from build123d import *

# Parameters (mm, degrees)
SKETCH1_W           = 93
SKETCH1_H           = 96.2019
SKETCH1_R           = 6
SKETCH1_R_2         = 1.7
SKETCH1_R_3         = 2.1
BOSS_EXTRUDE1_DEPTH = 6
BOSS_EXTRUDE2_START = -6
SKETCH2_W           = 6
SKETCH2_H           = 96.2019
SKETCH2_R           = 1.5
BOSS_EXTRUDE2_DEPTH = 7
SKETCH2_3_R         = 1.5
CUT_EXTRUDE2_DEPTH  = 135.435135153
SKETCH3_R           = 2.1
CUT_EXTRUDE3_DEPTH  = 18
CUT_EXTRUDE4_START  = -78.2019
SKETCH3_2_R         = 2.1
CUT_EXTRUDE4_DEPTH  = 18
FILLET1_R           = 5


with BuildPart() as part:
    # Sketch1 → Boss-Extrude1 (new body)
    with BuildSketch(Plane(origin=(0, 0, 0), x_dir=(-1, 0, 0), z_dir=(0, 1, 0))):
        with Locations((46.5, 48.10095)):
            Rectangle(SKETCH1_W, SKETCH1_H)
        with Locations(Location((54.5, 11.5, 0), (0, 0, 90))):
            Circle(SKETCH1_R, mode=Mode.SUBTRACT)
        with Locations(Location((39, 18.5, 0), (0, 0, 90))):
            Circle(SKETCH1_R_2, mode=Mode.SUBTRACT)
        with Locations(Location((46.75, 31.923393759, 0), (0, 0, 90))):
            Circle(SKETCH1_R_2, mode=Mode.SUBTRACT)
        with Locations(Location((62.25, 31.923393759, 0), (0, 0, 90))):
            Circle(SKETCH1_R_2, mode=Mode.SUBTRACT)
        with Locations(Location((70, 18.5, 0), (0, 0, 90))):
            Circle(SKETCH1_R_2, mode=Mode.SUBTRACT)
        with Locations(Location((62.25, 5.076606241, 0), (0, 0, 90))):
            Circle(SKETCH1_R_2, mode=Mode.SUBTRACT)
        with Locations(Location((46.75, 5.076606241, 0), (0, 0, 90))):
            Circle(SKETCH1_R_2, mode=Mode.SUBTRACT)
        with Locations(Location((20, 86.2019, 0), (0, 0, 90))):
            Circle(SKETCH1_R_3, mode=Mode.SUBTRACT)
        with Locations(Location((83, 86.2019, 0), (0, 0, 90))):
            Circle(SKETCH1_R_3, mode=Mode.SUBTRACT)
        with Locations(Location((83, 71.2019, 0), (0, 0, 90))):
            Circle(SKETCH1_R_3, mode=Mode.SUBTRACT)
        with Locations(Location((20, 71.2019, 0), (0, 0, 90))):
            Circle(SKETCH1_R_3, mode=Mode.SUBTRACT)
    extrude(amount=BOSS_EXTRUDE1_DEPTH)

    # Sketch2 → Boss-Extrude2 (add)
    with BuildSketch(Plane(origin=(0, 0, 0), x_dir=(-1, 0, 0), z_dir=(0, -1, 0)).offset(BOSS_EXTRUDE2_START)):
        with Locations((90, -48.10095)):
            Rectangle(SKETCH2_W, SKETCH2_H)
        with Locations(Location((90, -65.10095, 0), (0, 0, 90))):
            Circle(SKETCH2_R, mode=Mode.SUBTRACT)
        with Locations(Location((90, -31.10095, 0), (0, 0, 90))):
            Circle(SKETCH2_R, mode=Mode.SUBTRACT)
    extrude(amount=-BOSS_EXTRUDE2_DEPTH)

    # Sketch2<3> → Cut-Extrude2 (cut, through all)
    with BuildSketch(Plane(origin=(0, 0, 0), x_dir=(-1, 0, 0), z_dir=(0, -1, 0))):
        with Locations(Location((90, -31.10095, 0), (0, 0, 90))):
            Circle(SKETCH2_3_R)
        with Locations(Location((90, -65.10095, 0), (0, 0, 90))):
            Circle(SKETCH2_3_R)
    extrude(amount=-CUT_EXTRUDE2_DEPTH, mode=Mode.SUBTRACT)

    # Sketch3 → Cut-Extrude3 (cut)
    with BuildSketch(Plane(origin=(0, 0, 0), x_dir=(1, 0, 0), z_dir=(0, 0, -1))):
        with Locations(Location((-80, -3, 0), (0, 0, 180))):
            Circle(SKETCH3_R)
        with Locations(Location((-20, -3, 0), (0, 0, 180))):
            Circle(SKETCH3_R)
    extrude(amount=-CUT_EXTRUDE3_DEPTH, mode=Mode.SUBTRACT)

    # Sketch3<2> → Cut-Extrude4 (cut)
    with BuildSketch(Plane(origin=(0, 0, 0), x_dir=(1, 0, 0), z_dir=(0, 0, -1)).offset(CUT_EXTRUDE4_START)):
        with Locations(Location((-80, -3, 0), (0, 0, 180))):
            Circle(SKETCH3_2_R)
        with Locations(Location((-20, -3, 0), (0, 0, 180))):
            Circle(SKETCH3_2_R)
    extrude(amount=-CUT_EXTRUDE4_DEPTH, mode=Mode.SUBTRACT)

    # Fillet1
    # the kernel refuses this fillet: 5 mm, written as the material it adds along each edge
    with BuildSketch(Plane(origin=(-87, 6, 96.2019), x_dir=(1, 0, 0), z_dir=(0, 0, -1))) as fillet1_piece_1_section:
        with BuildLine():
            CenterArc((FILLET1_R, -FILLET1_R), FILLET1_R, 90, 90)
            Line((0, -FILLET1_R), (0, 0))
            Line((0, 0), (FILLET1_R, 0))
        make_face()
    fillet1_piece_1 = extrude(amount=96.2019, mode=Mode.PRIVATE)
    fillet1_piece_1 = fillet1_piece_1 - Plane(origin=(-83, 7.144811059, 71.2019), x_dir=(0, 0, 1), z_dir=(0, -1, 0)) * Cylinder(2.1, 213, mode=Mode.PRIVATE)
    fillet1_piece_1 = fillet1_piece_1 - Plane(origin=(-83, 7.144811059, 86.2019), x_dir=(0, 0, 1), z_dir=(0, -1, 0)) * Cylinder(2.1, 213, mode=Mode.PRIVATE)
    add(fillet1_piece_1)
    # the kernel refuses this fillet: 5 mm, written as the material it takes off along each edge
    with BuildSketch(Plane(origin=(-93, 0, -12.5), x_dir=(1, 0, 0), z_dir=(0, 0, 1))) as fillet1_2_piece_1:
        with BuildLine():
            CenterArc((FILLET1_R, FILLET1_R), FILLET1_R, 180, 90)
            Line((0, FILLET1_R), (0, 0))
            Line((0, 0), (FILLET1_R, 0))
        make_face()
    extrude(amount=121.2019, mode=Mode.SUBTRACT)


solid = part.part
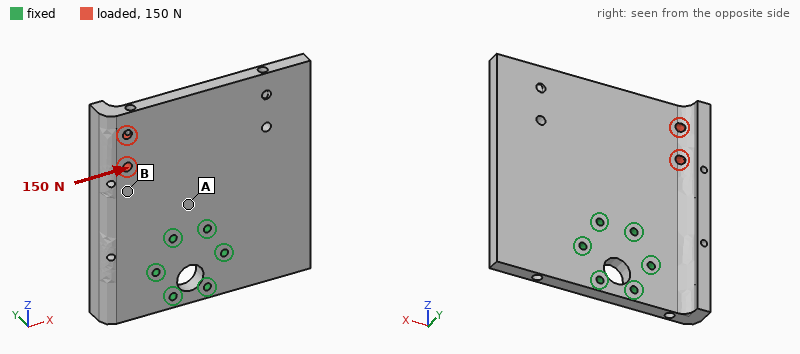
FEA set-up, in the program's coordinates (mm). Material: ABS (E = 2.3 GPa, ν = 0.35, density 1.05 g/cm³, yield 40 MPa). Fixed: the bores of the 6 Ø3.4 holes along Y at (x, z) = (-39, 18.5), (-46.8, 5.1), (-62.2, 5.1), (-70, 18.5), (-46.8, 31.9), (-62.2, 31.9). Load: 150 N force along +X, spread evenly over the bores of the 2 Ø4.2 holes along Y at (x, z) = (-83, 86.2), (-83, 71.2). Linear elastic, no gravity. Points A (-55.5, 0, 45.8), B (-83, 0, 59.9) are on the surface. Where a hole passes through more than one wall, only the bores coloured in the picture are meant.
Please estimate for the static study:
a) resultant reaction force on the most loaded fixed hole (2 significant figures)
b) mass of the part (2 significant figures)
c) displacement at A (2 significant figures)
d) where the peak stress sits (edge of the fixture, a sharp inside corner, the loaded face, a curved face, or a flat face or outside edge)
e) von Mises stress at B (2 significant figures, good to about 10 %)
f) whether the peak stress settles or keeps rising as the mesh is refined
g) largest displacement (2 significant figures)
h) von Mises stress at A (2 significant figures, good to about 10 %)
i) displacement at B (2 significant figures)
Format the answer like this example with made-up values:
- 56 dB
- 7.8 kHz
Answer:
- 140 N
- 58 g
- 18 µm
- edge of the fixture
- 0.55 MPa
- keeps rising
- 95 µm
- 1.2 MPa
- 46 µm
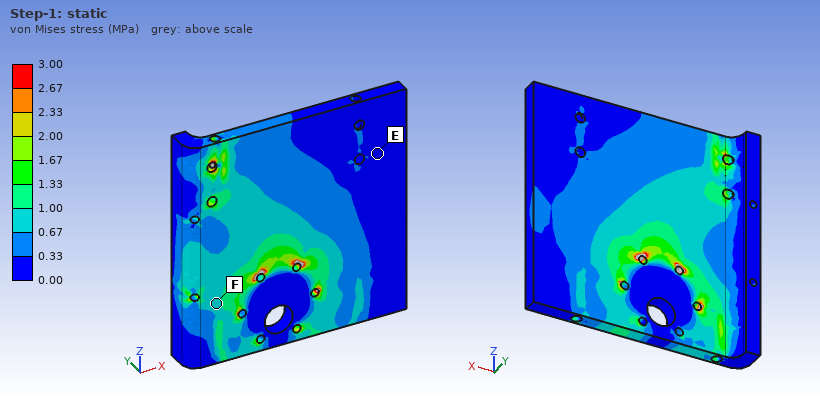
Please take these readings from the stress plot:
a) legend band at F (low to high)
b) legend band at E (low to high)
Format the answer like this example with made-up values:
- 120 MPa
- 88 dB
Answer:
- 0.67 to 1.00 MPa
- 0.00 to 0.33 MPa
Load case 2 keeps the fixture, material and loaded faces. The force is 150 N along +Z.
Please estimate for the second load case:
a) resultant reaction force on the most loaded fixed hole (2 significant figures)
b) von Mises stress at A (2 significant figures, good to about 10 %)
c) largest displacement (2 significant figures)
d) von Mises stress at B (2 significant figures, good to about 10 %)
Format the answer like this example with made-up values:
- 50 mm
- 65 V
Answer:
- 88 N
- 0.58 MPa
- 78 µm
- 1.2 MPa
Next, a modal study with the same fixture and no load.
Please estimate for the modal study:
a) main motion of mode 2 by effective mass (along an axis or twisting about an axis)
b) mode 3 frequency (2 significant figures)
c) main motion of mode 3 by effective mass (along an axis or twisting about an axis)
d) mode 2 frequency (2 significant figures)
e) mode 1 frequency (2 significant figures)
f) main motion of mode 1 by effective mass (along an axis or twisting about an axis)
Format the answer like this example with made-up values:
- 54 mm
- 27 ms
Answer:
- twisting about Z
- 890 Hz
- along Y
- 450 Hz
- 330 Hz
- along Y
